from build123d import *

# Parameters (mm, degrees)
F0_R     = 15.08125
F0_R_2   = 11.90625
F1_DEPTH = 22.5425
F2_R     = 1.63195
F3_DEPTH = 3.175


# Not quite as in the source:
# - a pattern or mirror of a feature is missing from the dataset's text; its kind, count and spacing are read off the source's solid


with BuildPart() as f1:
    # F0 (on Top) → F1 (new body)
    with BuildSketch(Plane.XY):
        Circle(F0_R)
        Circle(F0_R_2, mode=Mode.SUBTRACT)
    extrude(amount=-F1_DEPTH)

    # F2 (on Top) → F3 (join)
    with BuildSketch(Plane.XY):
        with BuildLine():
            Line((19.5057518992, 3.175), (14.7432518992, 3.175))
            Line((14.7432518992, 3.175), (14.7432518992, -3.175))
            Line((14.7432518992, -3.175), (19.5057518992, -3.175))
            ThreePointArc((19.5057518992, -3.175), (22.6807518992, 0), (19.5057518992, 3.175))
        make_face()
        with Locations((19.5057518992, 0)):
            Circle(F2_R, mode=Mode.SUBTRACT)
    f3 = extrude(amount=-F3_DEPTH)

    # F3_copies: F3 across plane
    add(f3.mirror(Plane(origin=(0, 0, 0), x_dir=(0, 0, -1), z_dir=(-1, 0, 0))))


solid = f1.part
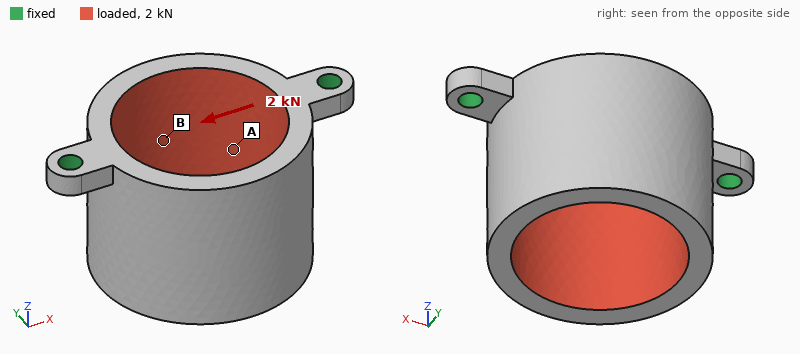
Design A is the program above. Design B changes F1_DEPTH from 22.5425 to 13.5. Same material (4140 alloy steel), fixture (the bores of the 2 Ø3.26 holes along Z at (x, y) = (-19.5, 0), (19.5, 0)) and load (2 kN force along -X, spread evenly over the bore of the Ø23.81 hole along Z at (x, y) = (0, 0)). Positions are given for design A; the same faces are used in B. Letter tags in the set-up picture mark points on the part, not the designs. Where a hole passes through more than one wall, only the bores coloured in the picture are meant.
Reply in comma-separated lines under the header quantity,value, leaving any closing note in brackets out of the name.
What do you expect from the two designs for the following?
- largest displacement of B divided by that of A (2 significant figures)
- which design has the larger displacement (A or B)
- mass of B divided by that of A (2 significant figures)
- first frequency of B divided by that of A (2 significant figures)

quantity,value
largest displacement of B divided by that of A,0.87
which design has the larger displacement,A
mass of B divided by that of A,0.61
first frequency of B divided by that of A,1.7
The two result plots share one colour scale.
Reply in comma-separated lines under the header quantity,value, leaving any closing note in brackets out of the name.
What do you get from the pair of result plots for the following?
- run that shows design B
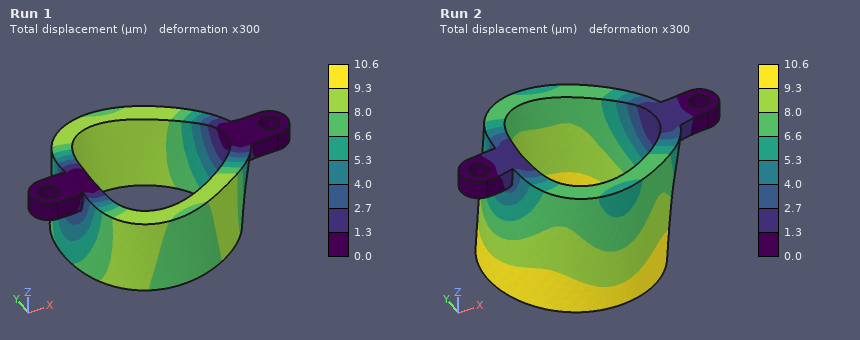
quantity,value
run that shows design B,Run 1
